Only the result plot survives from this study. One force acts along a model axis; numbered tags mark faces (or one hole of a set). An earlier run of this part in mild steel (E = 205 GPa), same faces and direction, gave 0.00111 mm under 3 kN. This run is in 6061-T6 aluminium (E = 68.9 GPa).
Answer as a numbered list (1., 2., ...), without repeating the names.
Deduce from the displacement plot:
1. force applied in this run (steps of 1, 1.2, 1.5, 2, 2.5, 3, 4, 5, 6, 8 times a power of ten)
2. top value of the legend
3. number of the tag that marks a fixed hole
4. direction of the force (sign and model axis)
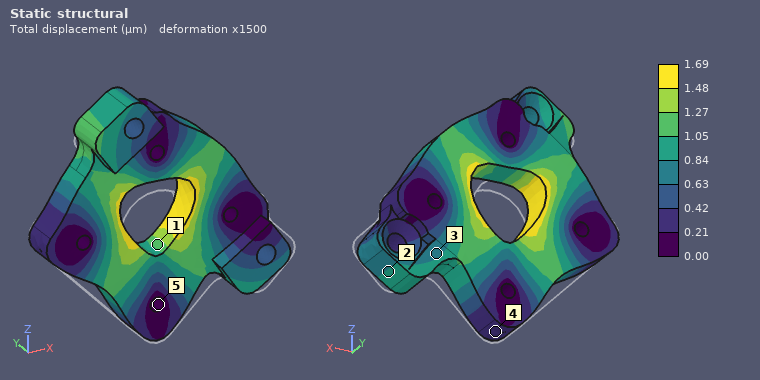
1. 1.5 kN
2. 1.69 µm
3. 5
4. +Z
